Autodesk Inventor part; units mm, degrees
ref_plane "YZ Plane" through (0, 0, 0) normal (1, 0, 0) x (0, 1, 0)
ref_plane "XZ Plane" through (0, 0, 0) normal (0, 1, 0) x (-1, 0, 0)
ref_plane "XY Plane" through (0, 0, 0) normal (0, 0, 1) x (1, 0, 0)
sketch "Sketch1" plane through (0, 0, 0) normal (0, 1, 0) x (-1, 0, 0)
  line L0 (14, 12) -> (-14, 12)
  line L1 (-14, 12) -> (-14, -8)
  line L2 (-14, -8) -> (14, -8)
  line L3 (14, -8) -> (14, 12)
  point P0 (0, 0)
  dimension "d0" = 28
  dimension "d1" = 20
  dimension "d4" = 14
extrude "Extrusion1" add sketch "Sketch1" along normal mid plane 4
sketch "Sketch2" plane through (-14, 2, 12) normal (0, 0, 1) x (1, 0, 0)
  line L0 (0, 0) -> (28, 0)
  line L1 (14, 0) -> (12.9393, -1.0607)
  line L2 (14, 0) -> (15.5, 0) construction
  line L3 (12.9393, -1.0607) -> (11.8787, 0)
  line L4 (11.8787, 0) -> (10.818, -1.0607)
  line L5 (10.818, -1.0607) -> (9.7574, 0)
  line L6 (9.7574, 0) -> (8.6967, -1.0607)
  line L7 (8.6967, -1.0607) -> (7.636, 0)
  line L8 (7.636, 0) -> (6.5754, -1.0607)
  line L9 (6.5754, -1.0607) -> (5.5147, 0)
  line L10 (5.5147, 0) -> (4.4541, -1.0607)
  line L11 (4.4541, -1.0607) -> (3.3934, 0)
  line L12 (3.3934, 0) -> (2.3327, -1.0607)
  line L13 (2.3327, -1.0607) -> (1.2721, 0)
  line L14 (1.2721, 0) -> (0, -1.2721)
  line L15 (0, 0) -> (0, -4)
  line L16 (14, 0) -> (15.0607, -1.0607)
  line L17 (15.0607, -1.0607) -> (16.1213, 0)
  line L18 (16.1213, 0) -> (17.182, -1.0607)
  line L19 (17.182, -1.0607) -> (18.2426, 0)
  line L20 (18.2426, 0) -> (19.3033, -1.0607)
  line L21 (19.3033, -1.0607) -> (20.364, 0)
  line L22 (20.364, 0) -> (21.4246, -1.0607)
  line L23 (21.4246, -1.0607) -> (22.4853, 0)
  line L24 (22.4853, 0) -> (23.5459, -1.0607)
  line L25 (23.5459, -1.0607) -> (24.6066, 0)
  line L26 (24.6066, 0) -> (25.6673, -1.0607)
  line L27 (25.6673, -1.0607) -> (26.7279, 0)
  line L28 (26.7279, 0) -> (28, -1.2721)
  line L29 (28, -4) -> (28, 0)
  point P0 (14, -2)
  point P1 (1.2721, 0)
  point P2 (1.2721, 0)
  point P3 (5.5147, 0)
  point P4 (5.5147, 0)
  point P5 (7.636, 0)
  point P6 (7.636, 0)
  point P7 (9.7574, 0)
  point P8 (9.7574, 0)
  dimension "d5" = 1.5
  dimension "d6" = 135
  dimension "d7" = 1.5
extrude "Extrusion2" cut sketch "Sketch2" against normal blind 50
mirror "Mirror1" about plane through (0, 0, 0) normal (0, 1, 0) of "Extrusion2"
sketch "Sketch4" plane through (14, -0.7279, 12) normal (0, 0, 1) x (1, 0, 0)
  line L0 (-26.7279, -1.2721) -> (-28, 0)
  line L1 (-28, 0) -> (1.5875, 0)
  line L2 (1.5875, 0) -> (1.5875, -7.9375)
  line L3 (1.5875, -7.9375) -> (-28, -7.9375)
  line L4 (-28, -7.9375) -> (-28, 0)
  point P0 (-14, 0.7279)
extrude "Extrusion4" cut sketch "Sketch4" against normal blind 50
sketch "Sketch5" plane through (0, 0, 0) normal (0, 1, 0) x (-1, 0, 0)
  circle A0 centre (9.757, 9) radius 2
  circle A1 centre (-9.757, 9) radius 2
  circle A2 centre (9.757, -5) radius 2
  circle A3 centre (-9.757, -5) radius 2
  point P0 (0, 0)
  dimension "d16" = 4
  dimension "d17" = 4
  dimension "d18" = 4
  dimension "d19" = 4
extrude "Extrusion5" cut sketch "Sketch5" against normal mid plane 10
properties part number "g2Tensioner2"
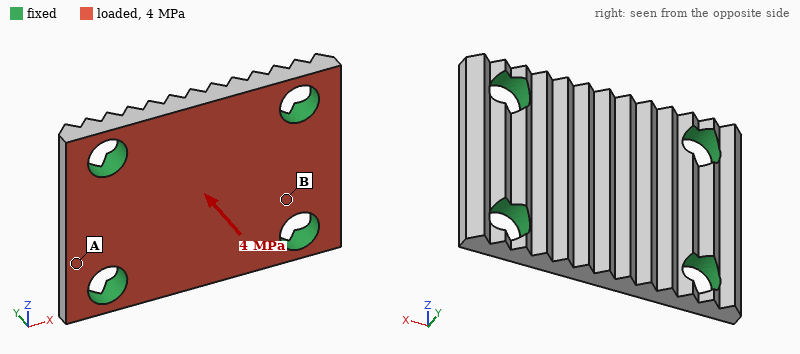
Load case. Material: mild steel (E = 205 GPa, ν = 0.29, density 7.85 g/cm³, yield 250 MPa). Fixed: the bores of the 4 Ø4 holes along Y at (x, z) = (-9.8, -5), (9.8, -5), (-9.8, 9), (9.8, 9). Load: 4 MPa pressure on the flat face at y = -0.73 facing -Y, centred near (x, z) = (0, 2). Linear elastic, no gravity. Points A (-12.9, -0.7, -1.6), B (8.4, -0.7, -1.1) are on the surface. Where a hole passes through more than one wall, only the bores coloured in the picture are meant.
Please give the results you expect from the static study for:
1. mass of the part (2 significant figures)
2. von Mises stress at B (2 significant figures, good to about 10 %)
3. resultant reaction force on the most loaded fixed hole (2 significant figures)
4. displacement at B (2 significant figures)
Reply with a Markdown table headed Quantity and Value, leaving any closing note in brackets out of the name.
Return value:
| Quantity | Value |
|---|---|
| mass of the part | 8.7 g |
| von Mises stress at B | 58 MPa |
| resultant reaction force on the most loaded fixed hole | 510 N |
| displacement at B | 1.6 µm |
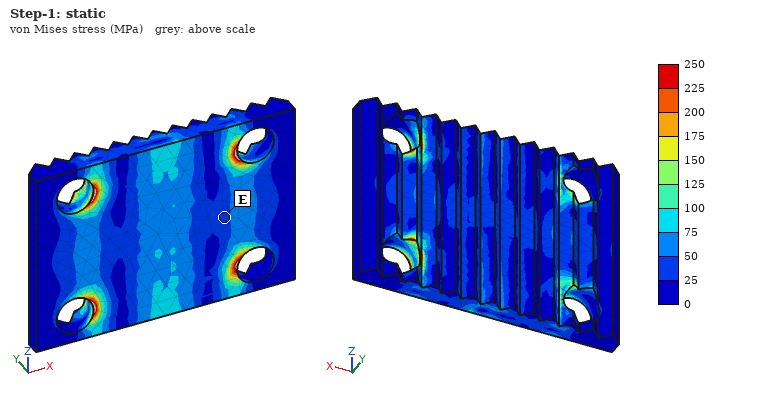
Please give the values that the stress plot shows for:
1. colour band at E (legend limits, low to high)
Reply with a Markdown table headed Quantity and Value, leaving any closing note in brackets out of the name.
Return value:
| Quantity | Value |
|---|---|
| colour band at E | 25 to 50 MPa |
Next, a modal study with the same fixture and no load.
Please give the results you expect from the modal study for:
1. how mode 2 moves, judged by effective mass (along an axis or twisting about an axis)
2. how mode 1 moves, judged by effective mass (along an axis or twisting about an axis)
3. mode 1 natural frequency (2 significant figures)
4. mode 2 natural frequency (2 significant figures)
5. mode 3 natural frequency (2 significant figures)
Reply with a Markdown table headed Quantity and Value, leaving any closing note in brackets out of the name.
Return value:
| Quantity | Value |
|---|---|
| how mode 2 moves, judged by effective mass | twisting about X |
| how mode 1 moves, judged by effective mass | along Y |
| mode 1 natural frequency | 29 kHz |
| mode 2 natural frequency | 37 kHz |
| mode 3 natural frequency | 51 kHz |
